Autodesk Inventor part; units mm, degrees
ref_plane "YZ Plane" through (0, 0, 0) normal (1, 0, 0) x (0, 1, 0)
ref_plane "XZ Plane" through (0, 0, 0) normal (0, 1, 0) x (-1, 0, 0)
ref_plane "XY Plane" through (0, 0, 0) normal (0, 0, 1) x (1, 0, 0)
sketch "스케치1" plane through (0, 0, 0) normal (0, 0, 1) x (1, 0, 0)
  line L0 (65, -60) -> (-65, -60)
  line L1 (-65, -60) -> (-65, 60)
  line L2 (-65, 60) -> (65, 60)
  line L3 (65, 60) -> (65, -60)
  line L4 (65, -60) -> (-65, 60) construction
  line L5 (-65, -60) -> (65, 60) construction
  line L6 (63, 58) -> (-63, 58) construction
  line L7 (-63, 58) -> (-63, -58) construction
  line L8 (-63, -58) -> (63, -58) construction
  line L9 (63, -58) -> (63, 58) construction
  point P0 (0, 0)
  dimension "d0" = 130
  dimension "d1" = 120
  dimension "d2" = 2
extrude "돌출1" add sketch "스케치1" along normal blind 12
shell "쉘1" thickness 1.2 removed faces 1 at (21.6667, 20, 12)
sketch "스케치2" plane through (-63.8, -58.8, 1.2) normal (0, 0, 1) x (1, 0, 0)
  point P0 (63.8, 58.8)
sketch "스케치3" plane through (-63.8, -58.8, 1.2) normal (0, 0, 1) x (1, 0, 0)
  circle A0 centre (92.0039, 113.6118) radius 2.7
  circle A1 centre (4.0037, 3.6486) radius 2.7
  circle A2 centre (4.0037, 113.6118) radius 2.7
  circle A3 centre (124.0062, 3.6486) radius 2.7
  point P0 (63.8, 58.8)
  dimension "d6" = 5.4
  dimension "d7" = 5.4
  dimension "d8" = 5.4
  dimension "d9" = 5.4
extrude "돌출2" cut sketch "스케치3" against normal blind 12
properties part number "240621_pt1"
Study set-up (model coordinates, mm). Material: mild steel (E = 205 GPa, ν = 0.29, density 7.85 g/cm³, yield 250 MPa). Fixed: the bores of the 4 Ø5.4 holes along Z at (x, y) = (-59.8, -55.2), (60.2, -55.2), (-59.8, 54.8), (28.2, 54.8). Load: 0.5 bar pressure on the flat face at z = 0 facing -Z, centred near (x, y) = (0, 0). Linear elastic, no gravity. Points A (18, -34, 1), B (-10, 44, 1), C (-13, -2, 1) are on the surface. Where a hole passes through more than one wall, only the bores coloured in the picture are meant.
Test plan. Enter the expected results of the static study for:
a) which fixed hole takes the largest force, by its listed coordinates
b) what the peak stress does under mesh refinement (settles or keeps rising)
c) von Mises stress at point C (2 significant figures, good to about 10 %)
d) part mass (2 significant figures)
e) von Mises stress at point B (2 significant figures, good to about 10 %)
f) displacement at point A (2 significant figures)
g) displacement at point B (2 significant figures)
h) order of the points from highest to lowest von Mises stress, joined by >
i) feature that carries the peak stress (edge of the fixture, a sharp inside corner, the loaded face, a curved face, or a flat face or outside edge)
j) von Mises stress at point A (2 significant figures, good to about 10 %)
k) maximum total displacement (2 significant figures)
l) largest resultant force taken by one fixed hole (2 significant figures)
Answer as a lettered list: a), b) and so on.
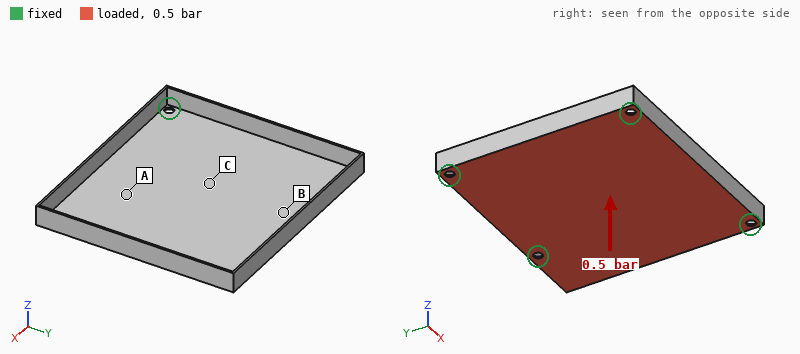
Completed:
a) (28.2, 54.8)
b) keeps rising
c) 100 MPa
d) 200 g
e) 36 MPa
f) 0.55 mm
g) 0.28 mm
h) C > A > B
i) edge of the fixture
j) 72 MPa
k) 0.91 mm
l) 280 N
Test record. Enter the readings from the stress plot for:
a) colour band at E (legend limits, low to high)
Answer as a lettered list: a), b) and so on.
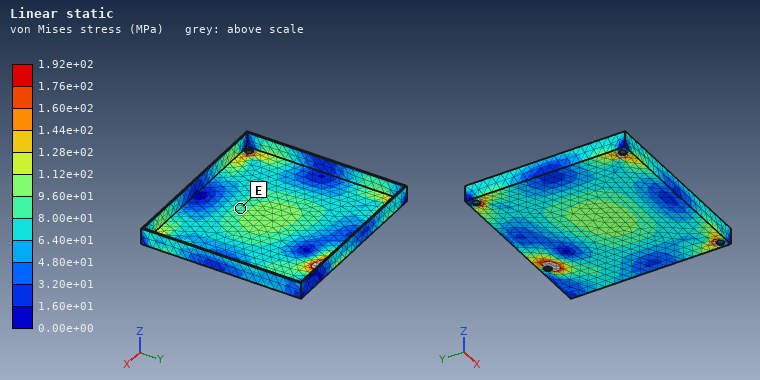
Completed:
a) 8.00e+01 to 9.60e+01 MPa
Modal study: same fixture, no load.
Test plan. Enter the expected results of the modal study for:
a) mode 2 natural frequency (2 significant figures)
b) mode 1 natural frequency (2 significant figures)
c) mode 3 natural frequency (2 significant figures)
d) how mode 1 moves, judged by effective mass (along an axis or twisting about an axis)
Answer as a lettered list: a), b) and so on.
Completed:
a) 980 Hz
b) 480 Hz
c) 1200 Hz
d) along Z
